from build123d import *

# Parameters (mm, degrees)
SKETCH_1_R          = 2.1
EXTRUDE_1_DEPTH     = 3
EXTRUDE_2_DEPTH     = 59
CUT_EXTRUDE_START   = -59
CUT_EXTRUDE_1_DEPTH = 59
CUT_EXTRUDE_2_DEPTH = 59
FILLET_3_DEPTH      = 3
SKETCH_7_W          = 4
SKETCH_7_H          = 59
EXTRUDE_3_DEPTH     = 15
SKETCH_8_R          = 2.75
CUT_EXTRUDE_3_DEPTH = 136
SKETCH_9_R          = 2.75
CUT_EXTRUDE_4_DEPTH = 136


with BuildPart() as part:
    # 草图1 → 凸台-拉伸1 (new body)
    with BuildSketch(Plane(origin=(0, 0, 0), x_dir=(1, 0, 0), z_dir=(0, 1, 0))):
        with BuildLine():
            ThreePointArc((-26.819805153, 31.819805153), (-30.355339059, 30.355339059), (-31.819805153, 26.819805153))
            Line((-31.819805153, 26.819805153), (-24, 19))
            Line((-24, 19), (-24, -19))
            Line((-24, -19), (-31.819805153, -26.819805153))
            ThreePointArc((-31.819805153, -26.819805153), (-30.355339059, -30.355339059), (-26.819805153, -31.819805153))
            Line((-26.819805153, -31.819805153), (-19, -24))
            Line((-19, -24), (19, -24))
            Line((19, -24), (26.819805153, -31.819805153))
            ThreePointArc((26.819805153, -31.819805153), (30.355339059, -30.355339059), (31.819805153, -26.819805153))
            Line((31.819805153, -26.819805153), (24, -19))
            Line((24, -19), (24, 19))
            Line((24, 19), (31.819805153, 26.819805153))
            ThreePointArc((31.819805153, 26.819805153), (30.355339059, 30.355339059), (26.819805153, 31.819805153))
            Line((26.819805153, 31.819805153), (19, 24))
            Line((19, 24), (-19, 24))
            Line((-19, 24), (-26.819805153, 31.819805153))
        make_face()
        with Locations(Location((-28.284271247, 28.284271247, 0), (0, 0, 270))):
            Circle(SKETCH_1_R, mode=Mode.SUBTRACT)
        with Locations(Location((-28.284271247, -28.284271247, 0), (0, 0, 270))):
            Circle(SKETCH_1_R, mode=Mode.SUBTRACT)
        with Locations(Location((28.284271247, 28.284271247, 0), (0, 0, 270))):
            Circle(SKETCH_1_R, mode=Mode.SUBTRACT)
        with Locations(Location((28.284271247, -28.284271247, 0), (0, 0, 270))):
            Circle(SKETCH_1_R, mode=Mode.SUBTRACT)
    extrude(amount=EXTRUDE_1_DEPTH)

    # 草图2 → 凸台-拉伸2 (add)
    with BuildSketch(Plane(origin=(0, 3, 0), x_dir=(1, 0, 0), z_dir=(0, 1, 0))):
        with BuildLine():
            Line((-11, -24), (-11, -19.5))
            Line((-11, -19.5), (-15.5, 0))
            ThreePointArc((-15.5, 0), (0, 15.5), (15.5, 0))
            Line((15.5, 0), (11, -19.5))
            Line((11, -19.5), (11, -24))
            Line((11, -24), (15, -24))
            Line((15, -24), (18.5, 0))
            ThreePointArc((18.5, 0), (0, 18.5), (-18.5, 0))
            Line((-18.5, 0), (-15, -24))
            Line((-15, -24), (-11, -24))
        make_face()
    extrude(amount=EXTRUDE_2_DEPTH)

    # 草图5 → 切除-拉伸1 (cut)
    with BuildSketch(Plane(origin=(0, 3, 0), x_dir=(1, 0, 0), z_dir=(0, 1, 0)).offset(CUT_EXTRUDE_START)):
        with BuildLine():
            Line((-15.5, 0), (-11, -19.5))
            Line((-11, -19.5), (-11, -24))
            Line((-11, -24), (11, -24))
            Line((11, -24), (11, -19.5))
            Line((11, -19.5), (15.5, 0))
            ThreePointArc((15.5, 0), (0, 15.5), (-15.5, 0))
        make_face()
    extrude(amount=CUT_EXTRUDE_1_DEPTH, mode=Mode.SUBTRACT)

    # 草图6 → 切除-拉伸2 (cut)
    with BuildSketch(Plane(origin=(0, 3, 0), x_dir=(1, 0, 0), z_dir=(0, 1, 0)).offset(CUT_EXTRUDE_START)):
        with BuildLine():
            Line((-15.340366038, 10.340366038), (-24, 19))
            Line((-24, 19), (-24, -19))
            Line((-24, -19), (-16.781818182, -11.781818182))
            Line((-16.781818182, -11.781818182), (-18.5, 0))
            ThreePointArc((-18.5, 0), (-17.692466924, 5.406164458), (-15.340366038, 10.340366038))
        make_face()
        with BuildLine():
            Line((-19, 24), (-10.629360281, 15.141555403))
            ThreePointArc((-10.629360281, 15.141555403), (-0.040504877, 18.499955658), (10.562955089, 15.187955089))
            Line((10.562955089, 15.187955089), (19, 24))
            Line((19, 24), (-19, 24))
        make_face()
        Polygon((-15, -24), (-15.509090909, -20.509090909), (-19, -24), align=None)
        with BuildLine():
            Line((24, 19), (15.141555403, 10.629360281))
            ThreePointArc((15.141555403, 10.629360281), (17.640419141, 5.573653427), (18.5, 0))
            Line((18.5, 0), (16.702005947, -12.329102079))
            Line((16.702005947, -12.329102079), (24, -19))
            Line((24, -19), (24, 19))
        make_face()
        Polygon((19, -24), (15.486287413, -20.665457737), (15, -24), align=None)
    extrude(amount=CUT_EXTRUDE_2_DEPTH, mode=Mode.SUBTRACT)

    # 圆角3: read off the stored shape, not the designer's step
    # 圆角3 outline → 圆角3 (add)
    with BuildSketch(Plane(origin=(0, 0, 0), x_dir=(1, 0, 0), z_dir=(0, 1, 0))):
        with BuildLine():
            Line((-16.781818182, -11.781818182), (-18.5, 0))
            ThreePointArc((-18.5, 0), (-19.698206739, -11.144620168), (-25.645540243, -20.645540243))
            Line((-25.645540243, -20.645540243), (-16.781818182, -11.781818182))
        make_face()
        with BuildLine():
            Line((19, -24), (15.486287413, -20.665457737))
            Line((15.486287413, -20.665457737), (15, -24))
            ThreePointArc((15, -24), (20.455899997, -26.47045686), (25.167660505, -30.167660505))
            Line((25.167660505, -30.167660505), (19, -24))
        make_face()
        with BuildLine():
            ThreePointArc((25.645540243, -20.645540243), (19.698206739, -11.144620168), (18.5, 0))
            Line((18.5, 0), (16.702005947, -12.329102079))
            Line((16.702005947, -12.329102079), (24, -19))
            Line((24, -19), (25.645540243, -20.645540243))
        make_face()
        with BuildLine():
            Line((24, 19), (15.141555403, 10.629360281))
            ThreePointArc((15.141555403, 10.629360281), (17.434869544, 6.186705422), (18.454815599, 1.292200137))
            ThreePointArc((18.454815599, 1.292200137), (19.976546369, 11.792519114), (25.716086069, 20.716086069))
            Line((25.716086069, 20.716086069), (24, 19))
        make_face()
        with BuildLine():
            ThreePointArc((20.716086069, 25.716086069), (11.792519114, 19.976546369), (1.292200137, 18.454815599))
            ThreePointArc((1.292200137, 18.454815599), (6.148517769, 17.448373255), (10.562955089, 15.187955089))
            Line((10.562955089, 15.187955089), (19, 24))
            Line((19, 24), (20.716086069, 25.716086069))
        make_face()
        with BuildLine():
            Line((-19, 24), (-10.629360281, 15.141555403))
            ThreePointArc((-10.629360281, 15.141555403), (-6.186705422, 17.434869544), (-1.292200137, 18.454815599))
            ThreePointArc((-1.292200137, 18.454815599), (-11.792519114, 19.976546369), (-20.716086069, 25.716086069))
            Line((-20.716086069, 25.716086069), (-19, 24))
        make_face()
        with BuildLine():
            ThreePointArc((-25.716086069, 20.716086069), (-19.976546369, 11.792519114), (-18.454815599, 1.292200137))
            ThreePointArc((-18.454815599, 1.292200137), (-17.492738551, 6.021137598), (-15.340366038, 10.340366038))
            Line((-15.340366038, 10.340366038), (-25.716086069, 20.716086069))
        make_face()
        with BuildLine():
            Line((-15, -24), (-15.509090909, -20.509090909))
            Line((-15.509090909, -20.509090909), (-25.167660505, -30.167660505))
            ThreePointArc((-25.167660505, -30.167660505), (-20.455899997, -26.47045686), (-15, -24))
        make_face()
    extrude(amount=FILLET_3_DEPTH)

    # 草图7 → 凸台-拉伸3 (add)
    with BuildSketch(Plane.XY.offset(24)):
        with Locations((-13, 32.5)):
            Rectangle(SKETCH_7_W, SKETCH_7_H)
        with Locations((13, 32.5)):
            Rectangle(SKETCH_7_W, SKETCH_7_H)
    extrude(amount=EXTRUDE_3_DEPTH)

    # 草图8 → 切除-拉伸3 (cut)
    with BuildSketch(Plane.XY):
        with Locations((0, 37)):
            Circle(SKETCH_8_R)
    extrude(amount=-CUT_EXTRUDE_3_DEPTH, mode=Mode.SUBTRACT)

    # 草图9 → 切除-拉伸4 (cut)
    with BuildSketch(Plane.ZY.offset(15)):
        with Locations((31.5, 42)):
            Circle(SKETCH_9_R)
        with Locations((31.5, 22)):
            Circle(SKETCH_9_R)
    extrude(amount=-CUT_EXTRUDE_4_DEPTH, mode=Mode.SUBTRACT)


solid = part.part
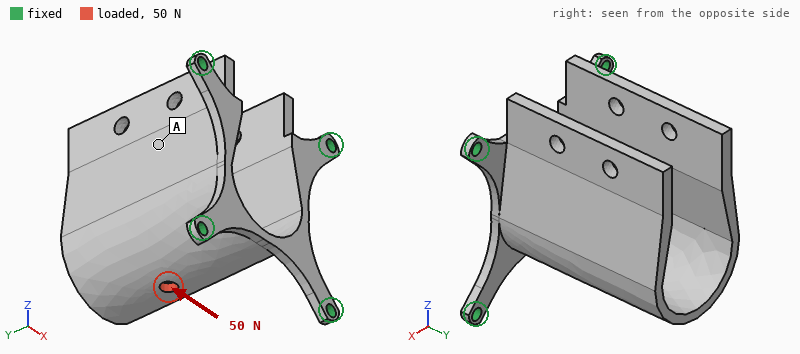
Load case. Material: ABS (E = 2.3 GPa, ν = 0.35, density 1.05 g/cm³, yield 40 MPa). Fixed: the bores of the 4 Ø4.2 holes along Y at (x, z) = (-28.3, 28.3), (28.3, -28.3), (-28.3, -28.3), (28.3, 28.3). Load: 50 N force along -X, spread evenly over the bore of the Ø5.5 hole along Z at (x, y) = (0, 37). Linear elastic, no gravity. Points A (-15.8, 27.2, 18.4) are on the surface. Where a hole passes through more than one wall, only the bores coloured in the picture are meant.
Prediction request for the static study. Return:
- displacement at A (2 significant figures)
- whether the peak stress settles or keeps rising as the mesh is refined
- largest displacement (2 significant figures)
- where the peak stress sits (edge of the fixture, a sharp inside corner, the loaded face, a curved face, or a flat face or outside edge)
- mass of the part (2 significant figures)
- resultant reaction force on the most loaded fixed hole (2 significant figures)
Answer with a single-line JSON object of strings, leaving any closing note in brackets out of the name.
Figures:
{"displacement at A": "0.45 mm", "whether the peak stress settles or keeps rising as the mesh is refined": "keeps rising", "largest displacement": "1.2 mm", "where the peak stress sits": "edge of the fixture", "mass of the part": "32 g", "resultant reaction force on the most loaded fixed hole": "31 N"}
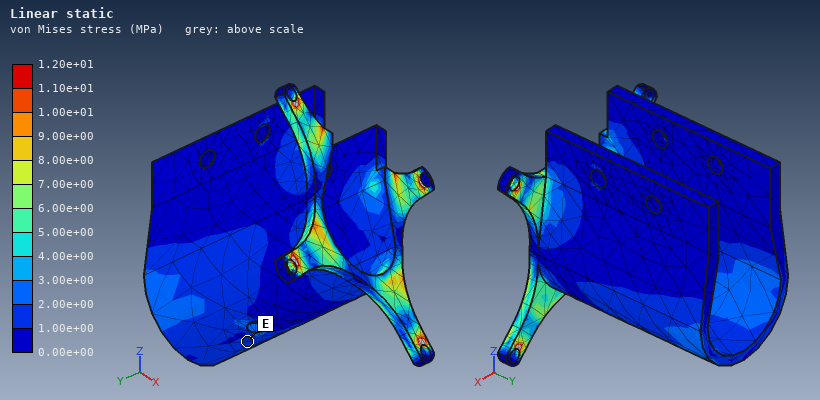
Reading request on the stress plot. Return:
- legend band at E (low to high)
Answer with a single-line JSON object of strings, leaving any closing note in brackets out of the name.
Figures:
{"legend band at E": "1.00e+00 to 2.00e+00 MPa"}
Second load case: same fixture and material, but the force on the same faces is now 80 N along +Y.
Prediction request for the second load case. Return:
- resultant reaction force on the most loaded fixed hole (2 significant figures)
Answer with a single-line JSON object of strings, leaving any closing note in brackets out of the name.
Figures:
{"resultant reaction force on the most loaded fixed hole": "40 N"}
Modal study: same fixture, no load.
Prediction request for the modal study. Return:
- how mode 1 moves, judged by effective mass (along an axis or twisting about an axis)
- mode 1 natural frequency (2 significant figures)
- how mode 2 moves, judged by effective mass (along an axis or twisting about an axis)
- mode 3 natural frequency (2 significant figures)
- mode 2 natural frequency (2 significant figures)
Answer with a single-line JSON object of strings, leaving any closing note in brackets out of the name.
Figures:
{"how mode 1 moves, judged by effective mass": "along X", "mode 1 natural frequency": "180 Hz", "how mode 2 moves, judged by effective mass": "along Z", "mode 3 natural frequency": "320 Hz", "mode 2 natural frequency": "270 Hz"}
